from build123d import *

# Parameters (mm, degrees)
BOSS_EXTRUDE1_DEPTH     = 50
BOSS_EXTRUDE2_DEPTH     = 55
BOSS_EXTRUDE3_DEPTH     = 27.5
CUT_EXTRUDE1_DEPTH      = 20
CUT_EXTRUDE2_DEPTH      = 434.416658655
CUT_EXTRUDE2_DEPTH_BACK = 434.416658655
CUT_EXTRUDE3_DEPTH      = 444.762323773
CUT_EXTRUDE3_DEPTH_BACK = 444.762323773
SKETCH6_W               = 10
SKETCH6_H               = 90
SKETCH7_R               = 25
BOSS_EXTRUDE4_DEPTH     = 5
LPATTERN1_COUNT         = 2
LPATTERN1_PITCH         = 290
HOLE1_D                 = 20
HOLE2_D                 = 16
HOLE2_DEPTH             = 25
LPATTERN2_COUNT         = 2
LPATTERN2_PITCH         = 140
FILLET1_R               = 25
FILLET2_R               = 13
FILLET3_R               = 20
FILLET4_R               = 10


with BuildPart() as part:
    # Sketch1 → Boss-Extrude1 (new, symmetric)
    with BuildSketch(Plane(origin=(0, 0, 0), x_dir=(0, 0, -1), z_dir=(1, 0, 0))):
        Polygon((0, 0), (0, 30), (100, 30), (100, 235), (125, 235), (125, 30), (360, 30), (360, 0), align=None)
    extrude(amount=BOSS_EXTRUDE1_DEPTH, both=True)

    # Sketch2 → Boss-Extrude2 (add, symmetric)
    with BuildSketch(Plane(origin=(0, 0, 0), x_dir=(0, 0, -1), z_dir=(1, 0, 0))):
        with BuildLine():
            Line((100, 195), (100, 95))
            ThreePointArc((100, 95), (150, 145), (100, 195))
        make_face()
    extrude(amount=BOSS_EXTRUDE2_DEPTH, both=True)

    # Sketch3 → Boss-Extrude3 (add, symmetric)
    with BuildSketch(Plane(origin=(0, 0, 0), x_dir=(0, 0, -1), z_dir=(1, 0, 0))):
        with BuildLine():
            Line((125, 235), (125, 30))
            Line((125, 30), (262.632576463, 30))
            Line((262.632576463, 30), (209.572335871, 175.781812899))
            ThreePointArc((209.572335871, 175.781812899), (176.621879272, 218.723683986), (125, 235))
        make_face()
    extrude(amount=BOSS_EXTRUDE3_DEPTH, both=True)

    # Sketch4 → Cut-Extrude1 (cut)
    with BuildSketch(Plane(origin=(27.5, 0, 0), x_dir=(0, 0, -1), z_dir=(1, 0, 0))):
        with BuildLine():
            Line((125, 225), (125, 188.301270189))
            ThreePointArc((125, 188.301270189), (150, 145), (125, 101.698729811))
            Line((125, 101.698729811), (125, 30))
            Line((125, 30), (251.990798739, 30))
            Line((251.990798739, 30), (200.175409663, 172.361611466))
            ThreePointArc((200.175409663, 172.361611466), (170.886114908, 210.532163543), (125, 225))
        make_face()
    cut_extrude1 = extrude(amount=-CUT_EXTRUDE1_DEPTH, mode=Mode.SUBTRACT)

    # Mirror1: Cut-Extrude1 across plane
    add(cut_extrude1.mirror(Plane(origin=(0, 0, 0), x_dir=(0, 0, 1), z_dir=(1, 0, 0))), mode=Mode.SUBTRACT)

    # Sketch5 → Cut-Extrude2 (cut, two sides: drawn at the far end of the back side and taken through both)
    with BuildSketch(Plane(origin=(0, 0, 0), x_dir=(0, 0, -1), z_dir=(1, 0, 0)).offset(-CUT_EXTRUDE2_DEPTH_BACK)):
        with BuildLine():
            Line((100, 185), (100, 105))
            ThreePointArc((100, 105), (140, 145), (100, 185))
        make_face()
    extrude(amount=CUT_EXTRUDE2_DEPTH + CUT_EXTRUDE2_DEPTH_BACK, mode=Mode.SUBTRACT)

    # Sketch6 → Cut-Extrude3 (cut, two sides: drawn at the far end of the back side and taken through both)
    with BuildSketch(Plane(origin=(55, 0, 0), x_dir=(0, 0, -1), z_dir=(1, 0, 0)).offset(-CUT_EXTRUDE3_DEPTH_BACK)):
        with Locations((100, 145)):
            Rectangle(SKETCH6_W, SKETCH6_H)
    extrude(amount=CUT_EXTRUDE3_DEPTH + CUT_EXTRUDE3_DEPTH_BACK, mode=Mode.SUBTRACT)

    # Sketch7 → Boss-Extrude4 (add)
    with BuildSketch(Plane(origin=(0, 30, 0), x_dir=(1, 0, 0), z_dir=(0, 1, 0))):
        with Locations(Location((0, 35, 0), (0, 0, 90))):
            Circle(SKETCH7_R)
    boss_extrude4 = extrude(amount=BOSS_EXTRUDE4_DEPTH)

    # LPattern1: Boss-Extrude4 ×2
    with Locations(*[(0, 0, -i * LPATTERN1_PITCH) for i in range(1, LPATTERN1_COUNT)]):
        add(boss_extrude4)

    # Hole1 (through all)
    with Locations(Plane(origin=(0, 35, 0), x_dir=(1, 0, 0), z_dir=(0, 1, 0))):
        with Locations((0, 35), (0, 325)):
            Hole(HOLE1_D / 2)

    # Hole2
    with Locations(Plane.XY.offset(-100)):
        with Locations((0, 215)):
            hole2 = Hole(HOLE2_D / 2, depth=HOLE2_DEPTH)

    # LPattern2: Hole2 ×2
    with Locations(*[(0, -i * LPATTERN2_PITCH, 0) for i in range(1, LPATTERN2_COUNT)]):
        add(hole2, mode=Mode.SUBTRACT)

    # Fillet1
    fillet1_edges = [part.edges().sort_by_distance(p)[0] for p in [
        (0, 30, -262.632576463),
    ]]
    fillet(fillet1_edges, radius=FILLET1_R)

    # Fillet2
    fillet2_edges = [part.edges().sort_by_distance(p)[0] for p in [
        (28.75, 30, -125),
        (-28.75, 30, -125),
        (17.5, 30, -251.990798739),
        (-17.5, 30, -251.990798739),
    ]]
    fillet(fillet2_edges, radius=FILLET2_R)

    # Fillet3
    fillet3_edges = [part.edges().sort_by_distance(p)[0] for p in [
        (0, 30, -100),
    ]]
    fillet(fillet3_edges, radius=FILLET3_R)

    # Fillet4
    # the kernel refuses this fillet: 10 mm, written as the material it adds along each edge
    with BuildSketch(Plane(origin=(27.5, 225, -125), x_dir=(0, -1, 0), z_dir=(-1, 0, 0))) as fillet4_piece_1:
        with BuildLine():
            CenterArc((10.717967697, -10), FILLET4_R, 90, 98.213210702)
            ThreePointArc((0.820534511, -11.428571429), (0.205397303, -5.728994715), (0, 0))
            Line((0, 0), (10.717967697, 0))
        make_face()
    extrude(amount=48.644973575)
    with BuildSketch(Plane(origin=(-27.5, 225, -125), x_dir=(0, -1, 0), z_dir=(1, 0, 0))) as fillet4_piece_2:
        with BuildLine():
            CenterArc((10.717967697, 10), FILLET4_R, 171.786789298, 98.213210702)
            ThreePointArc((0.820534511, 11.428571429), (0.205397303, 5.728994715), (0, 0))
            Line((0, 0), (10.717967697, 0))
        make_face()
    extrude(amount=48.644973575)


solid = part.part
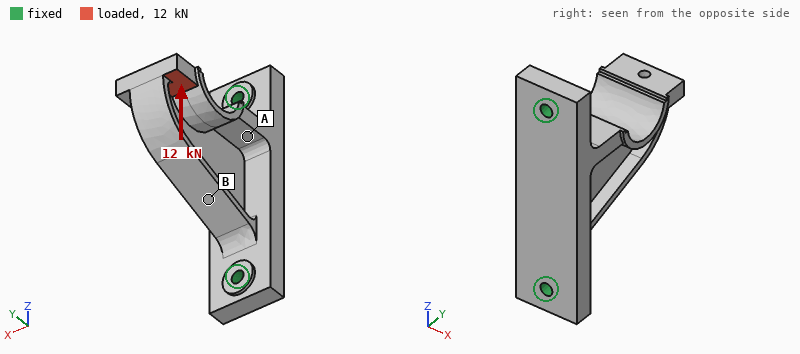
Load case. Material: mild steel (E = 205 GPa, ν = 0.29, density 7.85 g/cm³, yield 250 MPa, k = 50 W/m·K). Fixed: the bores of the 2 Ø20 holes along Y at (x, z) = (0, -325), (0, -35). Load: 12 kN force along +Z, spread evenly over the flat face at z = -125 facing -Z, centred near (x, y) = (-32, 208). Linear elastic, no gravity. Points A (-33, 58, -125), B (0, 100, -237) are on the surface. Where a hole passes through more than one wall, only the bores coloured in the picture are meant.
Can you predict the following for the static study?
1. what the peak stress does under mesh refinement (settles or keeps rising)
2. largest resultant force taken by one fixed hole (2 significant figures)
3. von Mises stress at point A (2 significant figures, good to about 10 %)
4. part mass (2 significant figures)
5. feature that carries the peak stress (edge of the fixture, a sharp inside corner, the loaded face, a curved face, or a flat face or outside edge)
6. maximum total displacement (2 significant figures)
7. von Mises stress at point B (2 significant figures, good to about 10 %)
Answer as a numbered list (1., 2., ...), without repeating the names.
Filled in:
1. keeps rising
2. 12 kN
3. 9.0 MPa
4. 15 kg
5. a sharp inside corner
6. 0.23 mm
7. 30 MPa
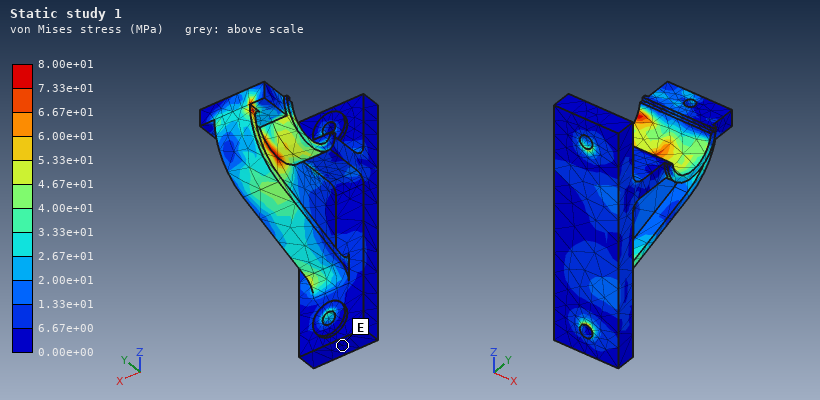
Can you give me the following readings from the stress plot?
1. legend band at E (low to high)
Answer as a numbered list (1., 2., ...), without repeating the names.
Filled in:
1. 0.00e+00 to 6.67e+00 MPa
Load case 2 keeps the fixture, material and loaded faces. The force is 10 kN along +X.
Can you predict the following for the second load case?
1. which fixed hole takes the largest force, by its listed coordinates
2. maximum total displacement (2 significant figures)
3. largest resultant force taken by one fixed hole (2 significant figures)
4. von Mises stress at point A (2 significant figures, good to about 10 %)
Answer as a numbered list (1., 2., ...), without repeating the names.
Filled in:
1. (0, -35)
2. 0.52 mm
3. 7.4 kN
4. 19 MPa
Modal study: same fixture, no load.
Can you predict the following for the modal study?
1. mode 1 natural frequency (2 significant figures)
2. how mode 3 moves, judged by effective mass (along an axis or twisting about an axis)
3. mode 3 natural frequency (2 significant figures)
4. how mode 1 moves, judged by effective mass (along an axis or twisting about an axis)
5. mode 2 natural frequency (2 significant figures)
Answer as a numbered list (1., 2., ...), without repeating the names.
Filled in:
1. 530 Hz
2. along Z
3. 1500 Hz
4. along X
5. 1200 Hz
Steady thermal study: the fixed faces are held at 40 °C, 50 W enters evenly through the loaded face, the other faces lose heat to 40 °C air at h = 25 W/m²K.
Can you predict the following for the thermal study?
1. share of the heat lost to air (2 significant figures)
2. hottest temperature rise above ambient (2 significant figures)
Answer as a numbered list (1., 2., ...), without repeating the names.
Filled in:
1. 84 %
2. 51 K
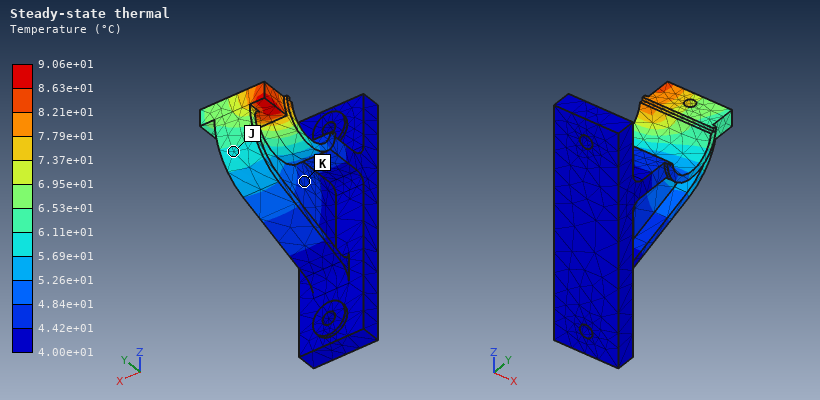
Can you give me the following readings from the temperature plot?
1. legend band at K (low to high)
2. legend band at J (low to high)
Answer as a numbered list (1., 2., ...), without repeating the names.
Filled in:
1. 4.42e+01 to 4.84e+01 °C
2. 5.69e+01 to 6.11e+01 °C
